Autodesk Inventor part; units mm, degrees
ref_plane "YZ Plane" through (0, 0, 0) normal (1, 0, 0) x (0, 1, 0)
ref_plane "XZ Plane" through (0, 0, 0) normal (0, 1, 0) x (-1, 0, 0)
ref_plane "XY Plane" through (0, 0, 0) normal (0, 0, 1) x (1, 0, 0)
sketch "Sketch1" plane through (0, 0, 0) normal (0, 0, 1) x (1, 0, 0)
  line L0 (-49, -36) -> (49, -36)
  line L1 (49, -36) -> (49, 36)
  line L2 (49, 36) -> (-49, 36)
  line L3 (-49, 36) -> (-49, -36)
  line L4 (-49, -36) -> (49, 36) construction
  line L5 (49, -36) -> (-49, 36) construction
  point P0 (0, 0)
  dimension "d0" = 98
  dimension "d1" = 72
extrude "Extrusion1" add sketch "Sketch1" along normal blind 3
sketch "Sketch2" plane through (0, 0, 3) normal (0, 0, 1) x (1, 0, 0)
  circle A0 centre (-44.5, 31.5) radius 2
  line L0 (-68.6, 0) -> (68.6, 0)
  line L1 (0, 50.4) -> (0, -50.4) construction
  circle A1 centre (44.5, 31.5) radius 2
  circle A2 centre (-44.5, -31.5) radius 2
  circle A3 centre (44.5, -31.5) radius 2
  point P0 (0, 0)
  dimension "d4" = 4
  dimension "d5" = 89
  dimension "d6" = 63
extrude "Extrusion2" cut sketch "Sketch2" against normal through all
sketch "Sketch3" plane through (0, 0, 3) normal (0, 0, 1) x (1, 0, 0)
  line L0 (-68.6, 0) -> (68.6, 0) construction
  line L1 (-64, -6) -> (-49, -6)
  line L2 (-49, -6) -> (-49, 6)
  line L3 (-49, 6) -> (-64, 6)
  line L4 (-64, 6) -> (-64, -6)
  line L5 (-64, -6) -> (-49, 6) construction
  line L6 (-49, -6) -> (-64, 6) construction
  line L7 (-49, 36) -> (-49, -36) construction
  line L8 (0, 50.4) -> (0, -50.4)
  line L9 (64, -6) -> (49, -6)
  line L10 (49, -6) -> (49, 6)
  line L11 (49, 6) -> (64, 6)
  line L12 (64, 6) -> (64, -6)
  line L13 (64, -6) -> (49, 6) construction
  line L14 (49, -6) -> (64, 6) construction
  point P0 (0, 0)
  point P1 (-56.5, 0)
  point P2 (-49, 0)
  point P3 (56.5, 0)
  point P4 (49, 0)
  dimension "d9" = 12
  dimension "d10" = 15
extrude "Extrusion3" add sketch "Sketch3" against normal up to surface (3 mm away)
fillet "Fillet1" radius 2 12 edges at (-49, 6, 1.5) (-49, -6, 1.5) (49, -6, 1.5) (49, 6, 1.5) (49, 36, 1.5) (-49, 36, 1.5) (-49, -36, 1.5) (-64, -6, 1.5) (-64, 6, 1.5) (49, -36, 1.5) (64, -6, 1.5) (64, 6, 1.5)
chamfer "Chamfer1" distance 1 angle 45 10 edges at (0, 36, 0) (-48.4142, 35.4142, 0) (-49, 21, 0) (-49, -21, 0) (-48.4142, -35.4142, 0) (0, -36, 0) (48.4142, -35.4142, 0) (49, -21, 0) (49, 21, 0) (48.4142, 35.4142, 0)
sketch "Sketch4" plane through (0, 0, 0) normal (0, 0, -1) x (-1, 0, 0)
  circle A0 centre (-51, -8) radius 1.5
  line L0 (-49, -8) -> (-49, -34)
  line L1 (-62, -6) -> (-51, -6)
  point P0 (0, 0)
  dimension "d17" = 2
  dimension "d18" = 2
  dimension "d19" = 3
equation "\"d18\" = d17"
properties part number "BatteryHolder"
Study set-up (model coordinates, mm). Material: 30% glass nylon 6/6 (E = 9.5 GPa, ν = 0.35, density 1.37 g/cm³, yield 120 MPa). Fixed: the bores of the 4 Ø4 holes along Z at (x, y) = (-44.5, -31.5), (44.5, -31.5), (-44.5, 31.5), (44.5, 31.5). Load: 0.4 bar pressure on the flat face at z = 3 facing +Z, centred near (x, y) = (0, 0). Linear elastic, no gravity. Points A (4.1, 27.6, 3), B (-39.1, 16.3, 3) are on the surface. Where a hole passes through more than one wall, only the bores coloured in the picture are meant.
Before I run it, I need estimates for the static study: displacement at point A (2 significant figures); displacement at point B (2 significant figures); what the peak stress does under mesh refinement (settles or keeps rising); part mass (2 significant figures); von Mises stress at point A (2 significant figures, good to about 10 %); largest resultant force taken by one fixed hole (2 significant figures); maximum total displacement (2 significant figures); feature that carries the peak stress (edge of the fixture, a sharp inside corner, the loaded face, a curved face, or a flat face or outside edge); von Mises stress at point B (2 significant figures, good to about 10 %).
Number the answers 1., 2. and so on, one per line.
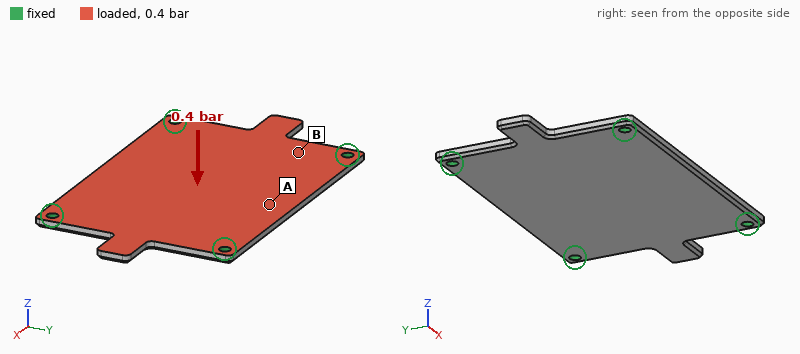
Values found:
1. 0.44 mm
2. 0.13 mm
3. keeps rising
4. 30 g
5. 11 MPa
6. 74 N
7. 0.50 mm
8. edge of the fixture
9. 5.3 MPa
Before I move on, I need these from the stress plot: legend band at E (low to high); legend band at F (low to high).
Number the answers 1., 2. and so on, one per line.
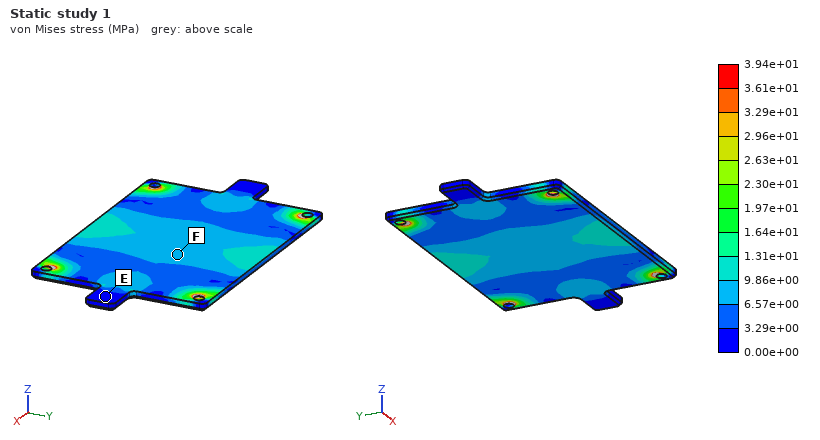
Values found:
1. 0.00e+00 to 3.29e+00 MPa
2. 6.57e+00 to 9.86e+00 MPa
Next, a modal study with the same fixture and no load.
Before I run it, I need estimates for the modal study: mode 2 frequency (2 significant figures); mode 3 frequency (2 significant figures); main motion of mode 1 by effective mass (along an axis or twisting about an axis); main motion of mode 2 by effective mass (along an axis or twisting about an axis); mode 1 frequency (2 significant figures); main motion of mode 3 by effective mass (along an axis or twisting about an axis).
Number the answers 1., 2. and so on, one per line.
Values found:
1. 1300 Hz
2. 1500 Hz
3. along Z
4. twisting about X
5. 810 Hz
6. along Z
